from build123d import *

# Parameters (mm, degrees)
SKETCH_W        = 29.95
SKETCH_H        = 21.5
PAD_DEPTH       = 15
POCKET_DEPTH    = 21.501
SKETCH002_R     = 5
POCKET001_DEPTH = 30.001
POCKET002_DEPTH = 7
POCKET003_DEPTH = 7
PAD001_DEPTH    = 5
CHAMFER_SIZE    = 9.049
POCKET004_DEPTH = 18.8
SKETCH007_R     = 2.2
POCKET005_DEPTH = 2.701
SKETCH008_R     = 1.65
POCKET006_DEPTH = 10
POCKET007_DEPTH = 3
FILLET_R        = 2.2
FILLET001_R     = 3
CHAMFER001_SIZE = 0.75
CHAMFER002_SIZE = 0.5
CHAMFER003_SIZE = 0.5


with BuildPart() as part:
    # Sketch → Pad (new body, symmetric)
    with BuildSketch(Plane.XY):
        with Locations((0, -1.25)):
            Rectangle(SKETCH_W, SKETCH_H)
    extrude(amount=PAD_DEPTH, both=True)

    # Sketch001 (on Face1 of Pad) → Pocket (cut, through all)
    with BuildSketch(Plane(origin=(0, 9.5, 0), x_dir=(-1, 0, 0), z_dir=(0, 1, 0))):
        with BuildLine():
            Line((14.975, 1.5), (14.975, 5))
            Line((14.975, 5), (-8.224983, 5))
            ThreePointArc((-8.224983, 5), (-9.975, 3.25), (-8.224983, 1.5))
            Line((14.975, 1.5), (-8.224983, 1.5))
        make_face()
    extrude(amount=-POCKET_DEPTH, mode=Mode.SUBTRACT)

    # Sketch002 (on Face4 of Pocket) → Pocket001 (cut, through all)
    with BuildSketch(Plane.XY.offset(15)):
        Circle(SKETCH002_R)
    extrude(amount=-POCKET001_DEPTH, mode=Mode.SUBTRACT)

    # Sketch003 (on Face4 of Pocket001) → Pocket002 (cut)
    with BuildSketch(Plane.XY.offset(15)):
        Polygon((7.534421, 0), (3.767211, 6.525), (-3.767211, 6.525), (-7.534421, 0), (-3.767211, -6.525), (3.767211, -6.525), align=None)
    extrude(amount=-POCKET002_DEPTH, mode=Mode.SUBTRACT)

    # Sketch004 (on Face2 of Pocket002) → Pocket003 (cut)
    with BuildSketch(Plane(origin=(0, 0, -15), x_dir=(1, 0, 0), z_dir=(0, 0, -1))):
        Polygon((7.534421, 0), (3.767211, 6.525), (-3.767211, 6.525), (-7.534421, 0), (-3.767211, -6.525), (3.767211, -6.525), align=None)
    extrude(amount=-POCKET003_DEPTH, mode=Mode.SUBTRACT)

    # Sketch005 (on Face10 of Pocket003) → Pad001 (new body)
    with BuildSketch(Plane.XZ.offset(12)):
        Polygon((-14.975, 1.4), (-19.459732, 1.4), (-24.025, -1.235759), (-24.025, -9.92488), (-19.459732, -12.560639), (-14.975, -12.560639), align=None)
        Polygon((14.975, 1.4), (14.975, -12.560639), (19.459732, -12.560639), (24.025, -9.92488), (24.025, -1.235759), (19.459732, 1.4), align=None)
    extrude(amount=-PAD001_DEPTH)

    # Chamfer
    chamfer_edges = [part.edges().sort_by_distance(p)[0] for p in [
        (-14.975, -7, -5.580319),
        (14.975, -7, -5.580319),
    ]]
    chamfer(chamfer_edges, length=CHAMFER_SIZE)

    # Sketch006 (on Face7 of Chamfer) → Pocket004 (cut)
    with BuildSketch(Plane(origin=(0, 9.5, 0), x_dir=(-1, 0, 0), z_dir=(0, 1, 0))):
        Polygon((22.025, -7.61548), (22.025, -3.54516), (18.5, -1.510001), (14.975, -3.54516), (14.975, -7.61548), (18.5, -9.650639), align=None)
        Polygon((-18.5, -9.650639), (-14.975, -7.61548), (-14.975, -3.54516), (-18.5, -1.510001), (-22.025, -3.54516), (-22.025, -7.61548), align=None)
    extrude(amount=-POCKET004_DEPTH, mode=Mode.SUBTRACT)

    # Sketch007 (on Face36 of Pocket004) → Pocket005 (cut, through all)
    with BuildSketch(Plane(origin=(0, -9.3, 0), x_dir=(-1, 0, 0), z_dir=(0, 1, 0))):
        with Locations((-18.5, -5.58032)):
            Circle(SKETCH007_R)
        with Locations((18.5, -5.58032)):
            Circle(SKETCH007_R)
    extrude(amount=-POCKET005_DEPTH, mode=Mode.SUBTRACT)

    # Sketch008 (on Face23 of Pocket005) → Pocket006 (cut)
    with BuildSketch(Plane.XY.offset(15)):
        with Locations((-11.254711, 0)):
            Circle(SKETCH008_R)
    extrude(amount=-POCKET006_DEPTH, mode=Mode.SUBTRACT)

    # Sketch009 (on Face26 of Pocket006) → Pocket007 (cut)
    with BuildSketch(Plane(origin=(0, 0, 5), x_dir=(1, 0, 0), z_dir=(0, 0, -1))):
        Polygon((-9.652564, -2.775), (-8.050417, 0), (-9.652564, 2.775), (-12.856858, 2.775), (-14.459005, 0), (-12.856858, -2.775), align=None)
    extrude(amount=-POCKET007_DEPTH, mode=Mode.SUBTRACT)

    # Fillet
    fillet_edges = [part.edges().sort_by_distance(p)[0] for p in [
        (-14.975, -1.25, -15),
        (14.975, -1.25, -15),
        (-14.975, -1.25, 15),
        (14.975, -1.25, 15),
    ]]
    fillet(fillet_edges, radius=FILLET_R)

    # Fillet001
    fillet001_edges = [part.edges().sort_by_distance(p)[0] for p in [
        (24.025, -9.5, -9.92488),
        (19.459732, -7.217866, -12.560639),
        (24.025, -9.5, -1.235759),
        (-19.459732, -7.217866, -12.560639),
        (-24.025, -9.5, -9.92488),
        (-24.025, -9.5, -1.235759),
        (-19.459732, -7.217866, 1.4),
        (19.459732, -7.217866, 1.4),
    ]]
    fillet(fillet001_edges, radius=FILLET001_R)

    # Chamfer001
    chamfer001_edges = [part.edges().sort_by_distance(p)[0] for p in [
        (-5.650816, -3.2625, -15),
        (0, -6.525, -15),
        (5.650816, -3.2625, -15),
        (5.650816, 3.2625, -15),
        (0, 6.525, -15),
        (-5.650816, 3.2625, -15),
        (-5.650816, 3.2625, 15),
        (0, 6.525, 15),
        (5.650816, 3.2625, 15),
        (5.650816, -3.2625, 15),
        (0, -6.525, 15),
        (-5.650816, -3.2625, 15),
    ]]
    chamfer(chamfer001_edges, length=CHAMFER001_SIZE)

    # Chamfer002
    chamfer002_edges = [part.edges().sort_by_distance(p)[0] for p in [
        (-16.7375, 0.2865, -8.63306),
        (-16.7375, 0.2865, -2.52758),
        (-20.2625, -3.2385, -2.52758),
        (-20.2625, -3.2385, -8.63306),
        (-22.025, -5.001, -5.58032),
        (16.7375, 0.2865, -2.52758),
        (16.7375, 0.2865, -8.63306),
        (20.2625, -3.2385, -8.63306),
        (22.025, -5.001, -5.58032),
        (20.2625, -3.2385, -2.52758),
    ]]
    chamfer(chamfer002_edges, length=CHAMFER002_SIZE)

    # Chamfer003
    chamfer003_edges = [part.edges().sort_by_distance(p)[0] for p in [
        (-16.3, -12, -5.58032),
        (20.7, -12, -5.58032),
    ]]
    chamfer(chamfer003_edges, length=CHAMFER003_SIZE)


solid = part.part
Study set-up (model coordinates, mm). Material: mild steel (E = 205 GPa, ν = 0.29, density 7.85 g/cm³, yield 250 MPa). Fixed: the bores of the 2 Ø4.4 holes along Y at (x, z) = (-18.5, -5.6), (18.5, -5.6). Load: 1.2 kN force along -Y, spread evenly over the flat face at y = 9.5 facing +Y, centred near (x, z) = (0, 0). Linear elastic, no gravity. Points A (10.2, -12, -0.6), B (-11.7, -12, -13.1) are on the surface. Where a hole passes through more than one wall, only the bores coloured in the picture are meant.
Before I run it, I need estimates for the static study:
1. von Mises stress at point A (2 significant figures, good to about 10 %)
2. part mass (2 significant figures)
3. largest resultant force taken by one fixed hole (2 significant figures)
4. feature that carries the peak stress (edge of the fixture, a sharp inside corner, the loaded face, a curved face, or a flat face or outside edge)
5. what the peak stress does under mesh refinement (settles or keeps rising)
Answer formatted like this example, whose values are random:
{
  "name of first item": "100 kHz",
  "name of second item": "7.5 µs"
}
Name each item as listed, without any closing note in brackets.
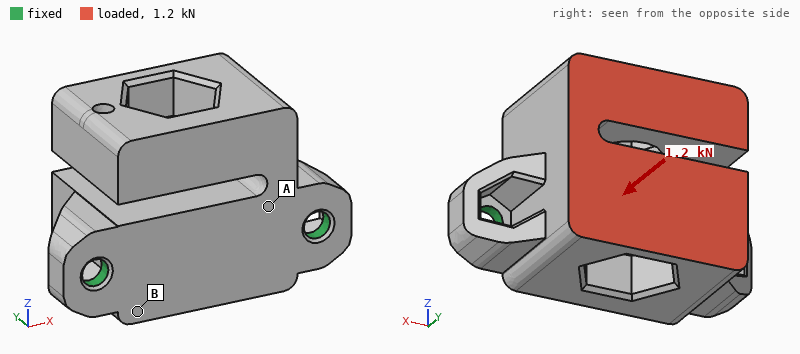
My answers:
{
  "von Mises stress at point A": "21 MPa",
  "part mass": "120 g",
  "largest resultant force taken by one fixed hole": "700 N",
  "feature that carries the peak stress": "edge of the fixture",
  "what the peak stress does under mesh refinement": "keeps rising"
}
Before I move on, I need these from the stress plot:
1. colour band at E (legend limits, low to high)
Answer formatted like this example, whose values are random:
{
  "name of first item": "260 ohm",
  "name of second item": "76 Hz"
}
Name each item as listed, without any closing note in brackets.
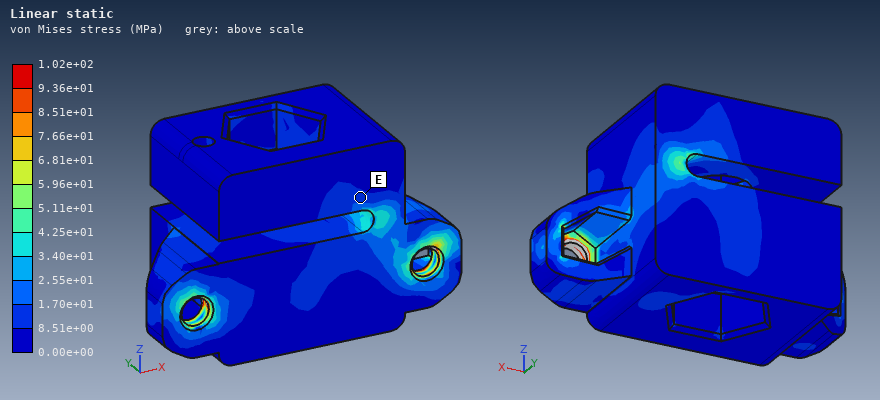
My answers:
{
  "colour band at E": "8.51e+00 to 1.70e+01 MPa"
}
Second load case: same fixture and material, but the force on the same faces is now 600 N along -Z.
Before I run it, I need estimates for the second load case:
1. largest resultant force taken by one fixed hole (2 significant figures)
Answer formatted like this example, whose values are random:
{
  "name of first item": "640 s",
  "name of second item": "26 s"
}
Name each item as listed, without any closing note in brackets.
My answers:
{
  "largest resultant force taken by one fixed hole": "310 N"
}
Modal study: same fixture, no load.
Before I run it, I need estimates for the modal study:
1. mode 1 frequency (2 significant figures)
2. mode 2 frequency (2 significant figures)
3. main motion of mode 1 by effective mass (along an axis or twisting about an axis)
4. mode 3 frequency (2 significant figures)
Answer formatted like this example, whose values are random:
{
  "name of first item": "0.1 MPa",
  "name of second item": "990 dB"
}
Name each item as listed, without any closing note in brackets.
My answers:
{
  "mode 1 frequency": "2900 Hz",
  "mode 2 frequency": "3700 Hz",
  "main motion of mode 1 by effective mass": "along Z",
  "mode 3 frequency": "7100 Hz"
}
